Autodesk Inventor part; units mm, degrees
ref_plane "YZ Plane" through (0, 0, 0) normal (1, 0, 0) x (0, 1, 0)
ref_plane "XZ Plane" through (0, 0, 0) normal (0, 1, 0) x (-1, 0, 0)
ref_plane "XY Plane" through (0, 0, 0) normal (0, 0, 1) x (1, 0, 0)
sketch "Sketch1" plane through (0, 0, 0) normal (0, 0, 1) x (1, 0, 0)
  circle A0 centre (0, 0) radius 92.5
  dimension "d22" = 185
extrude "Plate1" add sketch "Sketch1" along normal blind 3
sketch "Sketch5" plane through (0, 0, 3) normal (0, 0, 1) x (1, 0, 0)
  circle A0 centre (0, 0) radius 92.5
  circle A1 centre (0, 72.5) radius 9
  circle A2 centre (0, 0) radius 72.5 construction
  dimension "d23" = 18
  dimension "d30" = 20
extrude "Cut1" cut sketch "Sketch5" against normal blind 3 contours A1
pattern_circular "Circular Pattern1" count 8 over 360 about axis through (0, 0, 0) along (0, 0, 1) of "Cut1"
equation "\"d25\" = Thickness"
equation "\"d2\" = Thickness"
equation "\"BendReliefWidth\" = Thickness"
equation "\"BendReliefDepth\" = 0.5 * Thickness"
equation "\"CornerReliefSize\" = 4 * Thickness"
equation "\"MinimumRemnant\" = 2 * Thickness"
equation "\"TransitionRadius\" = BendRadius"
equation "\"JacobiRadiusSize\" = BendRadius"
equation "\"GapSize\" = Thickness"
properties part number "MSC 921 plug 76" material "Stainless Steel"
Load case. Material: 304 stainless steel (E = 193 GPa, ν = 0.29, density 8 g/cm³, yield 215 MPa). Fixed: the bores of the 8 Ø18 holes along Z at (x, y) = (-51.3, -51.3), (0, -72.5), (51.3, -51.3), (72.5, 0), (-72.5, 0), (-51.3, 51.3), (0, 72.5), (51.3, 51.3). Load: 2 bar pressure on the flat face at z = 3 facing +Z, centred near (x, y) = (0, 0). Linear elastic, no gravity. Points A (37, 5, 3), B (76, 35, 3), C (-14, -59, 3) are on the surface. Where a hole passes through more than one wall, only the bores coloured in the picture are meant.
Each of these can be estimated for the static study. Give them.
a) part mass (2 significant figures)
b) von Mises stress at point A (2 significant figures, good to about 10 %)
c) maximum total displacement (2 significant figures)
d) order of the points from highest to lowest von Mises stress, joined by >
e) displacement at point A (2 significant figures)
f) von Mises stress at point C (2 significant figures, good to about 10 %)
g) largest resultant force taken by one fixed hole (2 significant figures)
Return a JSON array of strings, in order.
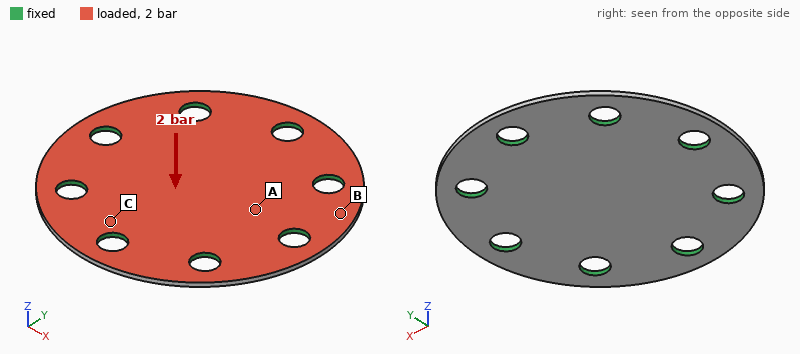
["600 g", "21 MPa", "0.13 mm", "C > A > B", "0.063 mm", "40 MPa", "620 N"]
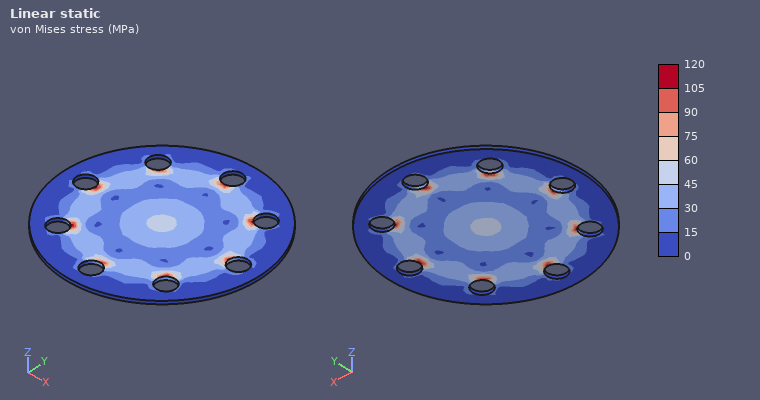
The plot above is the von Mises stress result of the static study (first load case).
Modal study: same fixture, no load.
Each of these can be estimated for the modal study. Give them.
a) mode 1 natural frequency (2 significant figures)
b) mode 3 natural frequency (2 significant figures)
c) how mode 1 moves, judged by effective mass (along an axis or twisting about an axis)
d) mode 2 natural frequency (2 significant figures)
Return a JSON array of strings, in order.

["1600 Hz", "3300 Hz", "along Z", "3300 Hz"]
